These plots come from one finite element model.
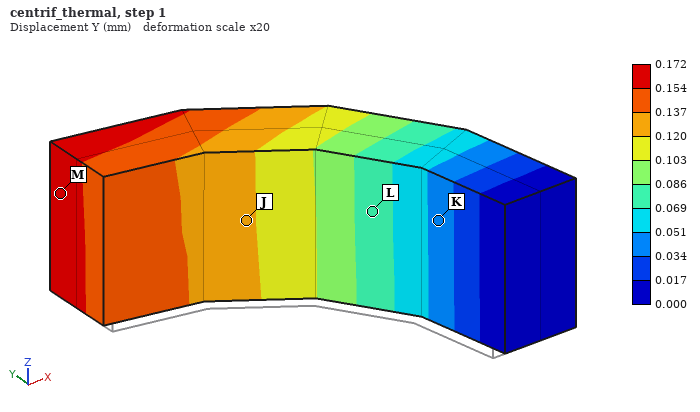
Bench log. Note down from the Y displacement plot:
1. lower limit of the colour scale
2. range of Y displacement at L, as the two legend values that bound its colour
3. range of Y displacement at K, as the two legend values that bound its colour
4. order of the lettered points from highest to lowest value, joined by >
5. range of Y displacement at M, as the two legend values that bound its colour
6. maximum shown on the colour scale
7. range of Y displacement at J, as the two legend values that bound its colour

0.000 mm
0.069 to 0.086 mm
0.034 to 0.051 mm
M > J > L > K
0.154 to 0.172 mm
0.172 mm
0.120 to 0.137 mm
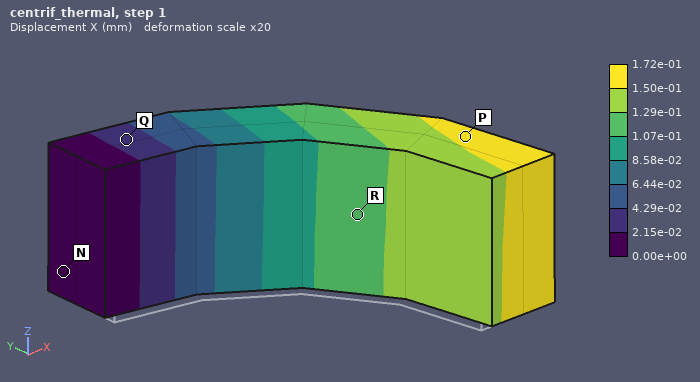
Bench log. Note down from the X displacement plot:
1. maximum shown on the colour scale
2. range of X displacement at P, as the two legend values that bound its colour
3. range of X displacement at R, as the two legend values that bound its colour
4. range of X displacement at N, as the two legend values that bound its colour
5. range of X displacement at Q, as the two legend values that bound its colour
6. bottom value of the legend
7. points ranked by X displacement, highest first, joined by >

1.72e-01 mm
1.50e-01 to 1.72e-01 mm
1.07e-01 to 1.29e-01 mm
0.00e+00 to 2.15e-02 mm
2.15e-02 to 4.29e-02 mm
0.00e+00 mm
P > R > Q > N
